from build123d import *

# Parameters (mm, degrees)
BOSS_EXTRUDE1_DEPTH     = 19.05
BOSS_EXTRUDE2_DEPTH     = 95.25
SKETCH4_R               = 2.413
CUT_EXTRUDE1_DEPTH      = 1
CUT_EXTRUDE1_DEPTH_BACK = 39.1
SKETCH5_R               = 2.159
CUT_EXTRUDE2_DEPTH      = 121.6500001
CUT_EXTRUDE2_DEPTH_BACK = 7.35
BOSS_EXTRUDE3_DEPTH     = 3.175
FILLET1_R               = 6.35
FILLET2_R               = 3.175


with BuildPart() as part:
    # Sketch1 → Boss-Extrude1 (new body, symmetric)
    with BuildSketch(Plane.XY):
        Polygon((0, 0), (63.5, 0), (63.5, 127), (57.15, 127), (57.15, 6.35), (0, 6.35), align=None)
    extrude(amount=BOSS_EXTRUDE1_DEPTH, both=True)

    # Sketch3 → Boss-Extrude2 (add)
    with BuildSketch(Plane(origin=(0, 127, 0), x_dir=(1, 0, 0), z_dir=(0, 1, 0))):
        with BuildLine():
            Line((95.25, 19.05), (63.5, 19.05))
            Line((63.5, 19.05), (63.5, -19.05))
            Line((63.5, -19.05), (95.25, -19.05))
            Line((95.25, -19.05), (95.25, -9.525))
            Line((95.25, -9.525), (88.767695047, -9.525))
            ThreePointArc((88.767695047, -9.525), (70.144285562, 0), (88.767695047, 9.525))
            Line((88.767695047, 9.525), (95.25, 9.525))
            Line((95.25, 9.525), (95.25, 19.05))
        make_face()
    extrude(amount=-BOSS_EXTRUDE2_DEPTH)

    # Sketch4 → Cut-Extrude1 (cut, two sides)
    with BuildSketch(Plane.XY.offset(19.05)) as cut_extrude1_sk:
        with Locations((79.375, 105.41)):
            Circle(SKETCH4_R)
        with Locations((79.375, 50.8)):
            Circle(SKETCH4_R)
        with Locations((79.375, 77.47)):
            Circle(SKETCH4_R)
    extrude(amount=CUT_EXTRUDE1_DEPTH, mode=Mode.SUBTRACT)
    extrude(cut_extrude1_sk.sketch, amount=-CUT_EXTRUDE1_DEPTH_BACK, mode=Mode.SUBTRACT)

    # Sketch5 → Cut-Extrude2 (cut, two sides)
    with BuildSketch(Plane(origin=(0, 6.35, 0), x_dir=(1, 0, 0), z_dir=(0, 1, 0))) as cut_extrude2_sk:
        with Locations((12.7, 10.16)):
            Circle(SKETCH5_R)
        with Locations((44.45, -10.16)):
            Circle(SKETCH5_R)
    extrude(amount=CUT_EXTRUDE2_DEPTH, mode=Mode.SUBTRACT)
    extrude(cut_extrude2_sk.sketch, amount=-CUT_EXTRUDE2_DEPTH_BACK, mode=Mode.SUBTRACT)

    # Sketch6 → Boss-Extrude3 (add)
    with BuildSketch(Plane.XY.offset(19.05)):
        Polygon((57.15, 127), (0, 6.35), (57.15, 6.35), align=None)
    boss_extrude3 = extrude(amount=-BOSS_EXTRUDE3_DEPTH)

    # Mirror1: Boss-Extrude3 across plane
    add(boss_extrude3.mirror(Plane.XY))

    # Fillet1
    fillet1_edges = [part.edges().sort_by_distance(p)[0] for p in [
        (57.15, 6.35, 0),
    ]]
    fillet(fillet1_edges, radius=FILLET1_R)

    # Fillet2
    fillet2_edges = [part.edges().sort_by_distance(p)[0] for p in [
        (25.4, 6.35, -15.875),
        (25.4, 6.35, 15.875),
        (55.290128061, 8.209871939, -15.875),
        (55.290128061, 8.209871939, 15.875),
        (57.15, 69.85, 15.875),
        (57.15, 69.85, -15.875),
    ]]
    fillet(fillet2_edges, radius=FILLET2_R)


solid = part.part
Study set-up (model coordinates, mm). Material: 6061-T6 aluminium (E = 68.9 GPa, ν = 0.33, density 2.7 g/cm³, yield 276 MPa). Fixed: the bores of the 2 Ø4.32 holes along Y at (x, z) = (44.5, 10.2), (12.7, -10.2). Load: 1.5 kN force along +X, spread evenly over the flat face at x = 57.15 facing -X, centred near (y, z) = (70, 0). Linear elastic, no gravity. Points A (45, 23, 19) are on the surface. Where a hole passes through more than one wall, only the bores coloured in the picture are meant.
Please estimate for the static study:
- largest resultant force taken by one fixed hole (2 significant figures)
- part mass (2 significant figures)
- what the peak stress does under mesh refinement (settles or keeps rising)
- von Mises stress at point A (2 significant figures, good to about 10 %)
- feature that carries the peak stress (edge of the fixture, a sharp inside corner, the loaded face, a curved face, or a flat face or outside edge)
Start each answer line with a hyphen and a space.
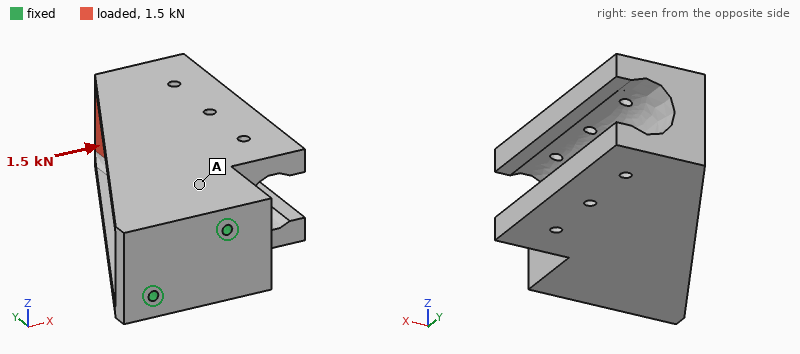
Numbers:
- 2.0 kN
- 360 g
- keeps rising
- 10 MPa
- edge of the fixture
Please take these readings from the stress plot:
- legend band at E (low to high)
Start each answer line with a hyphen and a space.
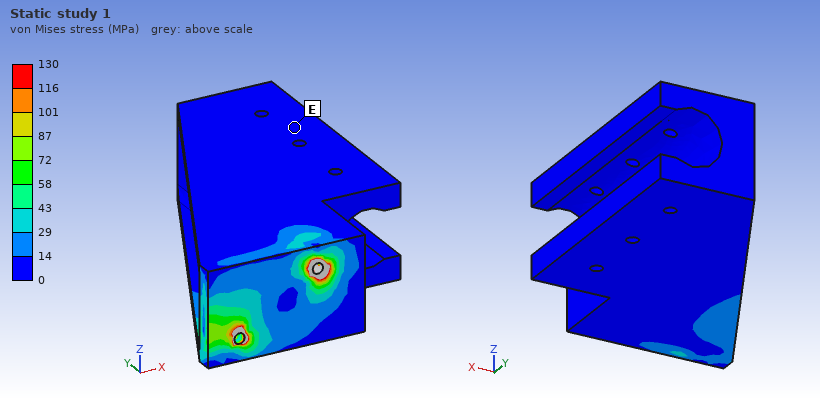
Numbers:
- 0 to 14 MPa
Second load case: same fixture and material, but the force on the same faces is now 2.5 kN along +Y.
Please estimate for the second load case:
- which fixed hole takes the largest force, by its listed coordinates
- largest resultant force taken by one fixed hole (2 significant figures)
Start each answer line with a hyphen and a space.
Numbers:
- (44.5, 10.2)
- 2.5 kN
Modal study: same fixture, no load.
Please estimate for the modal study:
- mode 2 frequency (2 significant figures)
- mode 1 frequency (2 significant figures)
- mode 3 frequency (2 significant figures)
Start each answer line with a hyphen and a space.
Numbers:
- 890 Hz
- 400 Hz
- 2000 Hz
